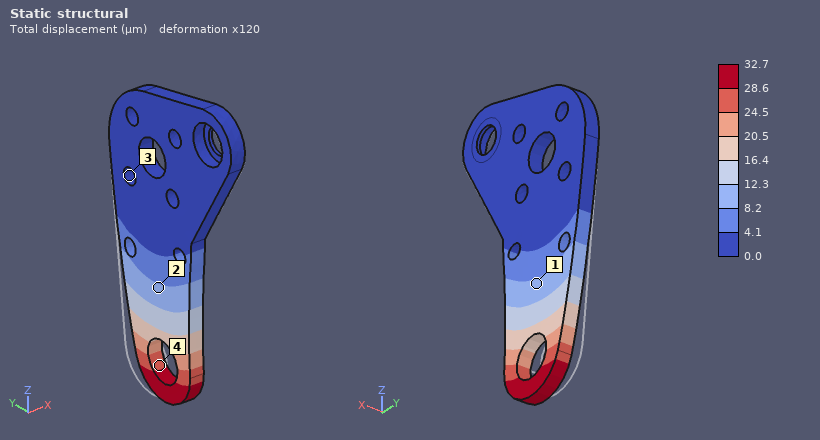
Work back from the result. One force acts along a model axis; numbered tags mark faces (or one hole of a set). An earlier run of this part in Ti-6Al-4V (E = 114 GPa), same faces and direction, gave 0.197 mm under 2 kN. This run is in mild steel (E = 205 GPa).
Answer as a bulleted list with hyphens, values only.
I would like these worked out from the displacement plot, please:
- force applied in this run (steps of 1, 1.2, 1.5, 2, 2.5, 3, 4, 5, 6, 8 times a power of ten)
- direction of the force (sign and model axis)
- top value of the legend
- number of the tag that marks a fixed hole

- 600 N
- -Y
- 32.7 µm
- 3
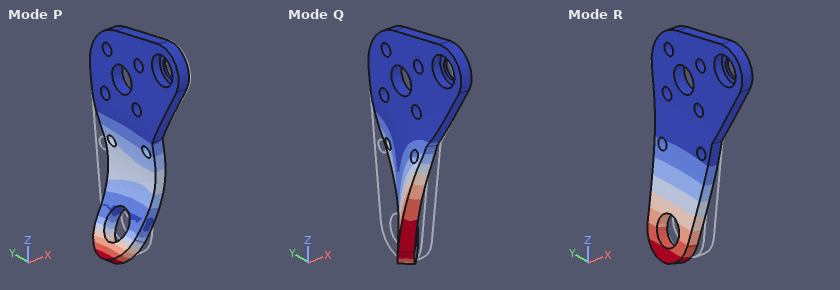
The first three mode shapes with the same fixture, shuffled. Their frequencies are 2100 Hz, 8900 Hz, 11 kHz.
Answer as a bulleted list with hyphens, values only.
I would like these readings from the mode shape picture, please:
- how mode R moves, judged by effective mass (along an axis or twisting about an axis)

- along X
